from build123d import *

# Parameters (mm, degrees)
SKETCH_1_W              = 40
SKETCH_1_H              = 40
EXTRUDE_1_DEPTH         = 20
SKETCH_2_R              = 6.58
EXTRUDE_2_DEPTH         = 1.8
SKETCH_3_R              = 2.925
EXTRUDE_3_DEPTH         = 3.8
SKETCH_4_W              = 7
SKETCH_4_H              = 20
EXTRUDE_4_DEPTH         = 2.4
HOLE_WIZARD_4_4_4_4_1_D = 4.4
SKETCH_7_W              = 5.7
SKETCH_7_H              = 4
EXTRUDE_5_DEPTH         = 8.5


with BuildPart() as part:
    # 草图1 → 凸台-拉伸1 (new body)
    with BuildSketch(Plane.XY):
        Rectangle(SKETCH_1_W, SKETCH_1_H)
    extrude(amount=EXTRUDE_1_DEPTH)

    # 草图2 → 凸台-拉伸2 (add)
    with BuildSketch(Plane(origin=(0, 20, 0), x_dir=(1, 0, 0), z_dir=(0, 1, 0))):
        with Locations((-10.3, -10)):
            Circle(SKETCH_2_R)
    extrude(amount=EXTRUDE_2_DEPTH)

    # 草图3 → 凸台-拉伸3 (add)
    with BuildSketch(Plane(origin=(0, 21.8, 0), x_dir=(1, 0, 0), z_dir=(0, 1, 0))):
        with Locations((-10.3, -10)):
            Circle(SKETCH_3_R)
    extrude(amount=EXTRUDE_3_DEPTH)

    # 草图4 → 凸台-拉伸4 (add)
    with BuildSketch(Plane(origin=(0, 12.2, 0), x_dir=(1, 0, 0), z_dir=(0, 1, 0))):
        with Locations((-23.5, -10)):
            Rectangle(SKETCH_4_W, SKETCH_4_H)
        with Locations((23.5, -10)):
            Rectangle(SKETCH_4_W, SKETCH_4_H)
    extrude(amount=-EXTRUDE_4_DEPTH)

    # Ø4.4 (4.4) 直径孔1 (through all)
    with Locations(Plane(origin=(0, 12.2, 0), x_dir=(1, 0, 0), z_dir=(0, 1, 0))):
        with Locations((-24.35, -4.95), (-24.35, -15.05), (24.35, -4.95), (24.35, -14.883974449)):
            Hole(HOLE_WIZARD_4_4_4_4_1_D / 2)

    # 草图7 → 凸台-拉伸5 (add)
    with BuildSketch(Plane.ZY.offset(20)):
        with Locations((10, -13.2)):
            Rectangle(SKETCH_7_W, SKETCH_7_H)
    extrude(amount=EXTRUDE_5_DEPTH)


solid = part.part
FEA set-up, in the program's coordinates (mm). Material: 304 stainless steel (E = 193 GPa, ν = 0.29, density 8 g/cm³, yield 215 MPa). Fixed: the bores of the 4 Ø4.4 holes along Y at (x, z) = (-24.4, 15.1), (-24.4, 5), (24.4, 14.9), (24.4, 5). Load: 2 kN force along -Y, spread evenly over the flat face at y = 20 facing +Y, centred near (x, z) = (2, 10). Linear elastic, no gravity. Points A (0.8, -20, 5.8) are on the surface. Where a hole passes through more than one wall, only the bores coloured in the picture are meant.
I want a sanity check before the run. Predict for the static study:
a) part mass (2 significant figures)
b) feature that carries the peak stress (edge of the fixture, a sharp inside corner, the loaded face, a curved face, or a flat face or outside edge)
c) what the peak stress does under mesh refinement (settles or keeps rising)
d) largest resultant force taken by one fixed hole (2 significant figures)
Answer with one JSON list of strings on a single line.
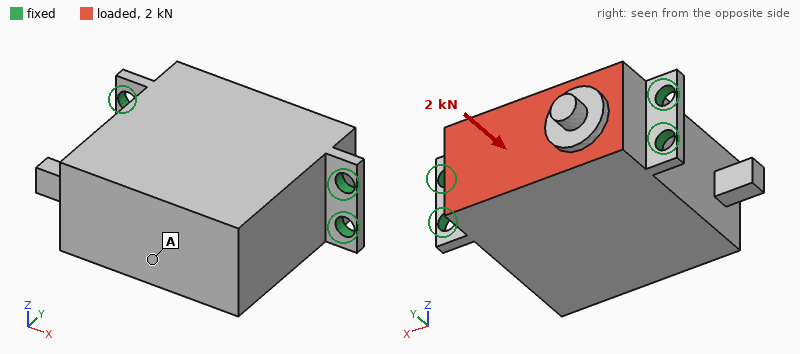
["260 g", "edge of the fixture", "keeps rising", "550 N"]
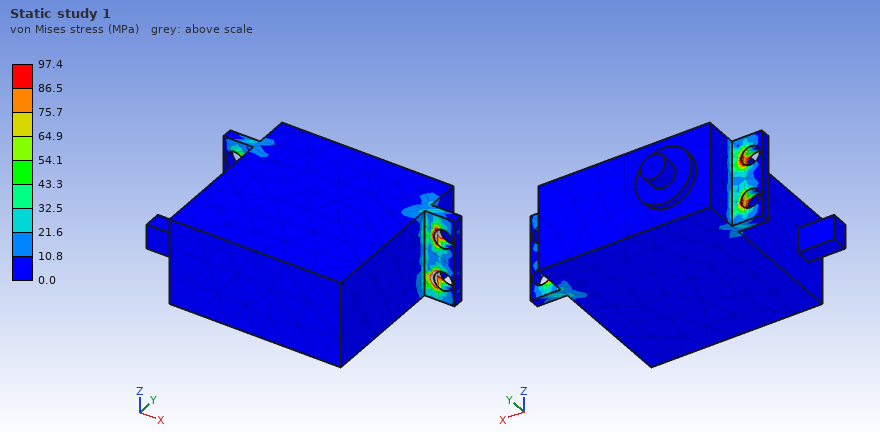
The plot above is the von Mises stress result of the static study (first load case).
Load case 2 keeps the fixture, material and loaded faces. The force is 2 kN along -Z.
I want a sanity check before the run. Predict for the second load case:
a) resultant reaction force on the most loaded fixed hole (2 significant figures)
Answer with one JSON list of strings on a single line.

["940 N"]
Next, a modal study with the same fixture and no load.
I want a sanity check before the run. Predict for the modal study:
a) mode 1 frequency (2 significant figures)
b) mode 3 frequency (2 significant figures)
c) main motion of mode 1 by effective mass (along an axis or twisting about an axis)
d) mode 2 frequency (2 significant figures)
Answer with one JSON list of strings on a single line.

["3000 Hz", "8800 Hz", "along Z", "8700 Hz"]
